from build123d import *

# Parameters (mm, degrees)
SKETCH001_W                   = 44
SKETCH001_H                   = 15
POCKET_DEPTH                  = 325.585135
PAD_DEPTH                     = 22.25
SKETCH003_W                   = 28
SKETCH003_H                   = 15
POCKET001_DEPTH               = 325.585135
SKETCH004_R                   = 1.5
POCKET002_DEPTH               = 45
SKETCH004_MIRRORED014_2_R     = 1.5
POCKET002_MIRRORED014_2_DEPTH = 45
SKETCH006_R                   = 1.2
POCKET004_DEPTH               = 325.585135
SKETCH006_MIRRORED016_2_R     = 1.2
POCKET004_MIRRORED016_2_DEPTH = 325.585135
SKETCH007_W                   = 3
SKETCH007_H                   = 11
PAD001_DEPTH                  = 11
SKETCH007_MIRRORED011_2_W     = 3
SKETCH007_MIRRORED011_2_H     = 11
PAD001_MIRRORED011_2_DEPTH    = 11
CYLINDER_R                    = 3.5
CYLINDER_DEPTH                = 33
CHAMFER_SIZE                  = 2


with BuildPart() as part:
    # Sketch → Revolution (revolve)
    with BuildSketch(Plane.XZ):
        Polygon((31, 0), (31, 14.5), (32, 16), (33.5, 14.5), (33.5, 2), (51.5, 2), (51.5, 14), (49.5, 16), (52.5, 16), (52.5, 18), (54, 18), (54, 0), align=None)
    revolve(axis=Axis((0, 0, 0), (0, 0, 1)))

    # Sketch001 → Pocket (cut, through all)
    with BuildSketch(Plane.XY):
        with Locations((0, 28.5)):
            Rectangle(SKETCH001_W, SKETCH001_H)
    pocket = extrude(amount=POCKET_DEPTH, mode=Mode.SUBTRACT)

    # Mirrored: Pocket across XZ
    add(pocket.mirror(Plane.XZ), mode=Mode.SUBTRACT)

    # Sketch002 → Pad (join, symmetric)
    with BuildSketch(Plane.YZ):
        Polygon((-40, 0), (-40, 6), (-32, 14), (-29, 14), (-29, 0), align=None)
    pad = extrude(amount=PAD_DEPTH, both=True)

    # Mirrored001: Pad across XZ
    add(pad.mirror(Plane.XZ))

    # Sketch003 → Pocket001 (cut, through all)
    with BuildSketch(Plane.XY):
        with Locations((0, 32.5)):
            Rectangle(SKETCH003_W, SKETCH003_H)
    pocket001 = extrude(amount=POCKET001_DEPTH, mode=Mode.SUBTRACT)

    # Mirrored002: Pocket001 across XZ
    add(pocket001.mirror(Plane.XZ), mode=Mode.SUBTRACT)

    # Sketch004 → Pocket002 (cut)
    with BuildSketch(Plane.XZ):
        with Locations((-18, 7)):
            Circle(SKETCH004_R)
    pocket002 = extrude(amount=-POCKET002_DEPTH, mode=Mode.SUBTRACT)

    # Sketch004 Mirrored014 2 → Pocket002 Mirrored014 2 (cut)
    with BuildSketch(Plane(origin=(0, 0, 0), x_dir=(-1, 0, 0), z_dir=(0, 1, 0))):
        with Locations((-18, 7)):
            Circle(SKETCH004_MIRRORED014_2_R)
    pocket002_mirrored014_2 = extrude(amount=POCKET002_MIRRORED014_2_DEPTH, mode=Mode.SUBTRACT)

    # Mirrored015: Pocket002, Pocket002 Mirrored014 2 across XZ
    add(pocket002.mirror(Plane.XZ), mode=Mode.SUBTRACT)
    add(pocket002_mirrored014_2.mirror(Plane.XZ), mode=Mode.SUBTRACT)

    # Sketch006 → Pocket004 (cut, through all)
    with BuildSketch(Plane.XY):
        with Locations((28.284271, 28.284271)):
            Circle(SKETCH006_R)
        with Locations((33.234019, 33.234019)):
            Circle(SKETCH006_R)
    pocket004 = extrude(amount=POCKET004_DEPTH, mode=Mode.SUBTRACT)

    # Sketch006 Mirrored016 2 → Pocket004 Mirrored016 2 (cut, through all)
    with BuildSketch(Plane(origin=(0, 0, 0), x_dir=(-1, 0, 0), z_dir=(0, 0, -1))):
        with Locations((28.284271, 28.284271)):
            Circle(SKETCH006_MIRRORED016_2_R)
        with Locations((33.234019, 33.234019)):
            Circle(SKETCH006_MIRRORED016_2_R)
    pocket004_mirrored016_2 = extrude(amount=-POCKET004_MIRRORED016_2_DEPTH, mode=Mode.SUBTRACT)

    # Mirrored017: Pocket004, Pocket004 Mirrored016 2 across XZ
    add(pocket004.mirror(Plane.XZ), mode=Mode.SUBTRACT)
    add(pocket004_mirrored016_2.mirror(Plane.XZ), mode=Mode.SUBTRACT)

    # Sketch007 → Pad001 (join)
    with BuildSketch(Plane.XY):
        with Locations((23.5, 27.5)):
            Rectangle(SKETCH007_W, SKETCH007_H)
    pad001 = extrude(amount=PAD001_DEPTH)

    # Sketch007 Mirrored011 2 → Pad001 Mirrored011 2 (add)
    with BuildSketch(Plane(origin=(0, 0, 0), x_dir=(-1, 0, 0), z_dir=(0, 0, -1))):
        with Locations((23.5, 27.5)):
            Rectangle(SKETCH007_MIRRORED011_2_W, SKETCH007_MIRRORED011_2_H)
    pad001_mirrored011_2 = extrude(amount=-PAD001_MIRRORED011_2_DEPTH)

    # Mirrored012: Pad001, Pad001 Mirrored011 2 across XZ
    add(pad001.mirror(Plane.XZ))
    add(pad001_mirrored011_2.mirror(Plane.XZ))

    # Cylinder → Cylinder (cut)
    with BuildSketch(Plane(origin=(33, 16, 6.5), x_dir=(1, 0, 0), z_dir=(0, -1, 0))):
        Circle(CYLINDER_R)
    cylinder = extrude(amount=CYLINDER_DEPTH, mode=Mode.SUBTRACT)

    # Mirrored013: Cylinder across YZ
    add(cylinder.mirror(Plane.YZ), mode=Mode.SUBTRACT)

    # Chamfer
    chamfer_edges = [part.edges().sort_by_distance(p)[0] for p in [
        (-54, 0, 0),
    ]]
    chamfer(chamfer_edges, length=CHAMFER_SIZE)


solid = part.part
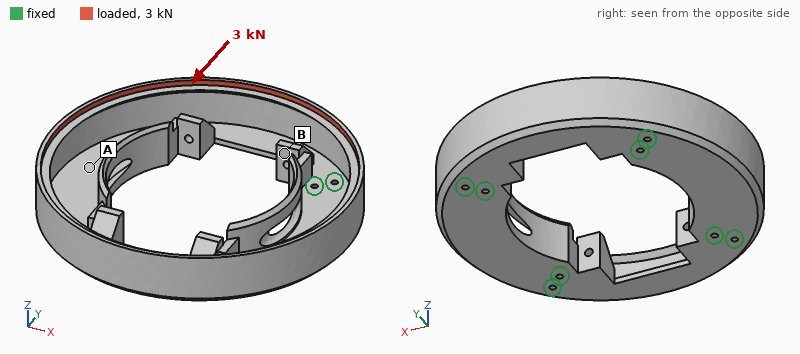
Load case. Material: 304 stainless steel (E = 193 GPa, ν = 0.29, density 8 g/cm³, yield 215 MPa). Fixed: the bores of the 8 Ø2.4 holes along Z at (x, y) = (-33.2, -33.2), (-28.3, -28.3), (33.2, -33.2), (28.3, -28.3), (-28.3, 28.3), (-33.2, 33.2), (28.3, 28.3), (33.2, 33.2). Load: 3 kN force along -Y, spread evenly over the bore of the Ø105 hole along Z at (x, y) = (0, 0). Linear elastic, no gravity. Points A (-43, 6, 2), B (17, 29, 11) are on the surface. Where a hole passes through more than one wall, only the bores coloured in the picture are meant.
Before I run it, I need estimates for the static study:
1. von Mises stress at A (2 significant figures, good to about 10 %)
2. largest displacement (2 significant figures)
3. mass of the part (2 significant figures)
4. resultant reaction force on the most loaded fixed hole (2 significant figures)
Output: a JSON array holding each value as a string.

["16 MPa", "40 µm", "240 g", "750 N"]
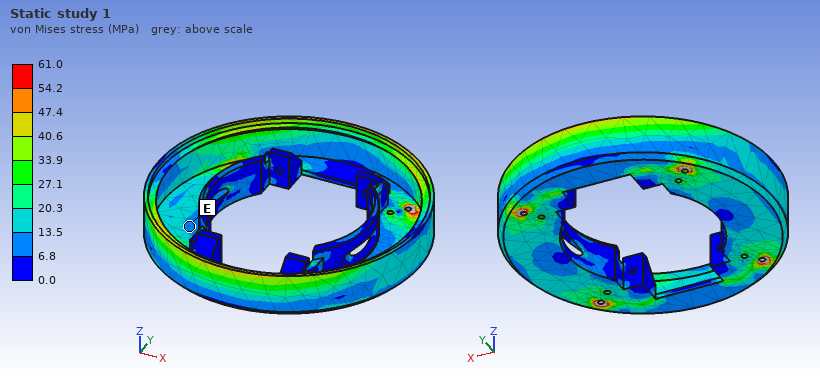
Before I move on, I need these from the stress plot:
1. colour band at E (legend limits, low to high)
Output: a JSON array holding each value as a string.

["6.8 to 13.5 MPa"]
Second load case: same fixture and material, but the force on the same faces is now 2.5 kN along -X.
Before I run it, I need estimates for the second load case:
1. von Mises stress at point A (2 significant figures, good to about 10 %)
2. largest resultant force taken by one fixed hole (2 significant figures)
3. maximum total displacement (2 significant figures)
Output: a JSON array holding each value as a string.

["10 MPa", "720 N", "38 µm"]
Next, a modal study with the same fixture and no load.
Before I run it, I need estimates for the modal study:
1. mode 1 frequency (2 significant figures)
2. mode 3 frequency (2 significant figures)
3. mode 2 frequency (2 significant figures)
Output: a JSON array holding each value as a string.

["1900 Hz", "3700 Hz", "3500 Hz"]
